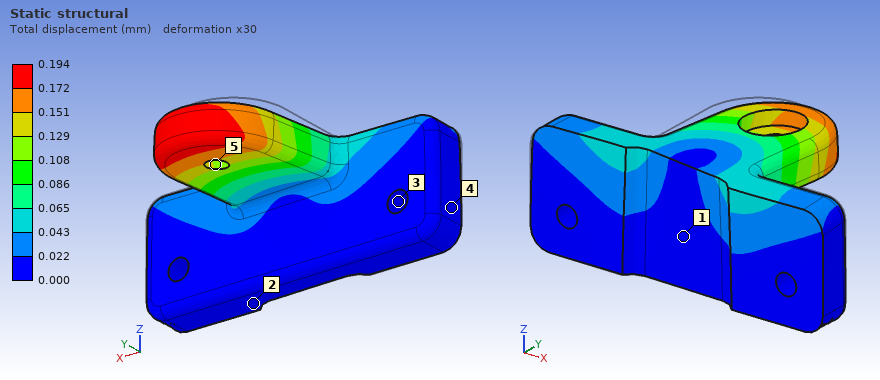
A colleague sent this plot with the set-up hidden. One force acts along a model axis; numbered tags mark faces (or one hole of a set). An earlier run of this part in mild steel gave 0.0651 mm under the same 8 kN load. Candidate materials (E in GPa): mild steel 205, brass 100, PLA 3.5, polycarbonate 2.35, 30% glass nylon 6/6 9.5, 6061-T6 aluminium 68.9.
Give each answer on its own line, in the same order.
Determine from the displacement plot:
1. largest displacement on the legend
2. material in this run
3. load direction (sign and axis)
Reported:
0.194 mm
6061-T6 aluminium
+X
